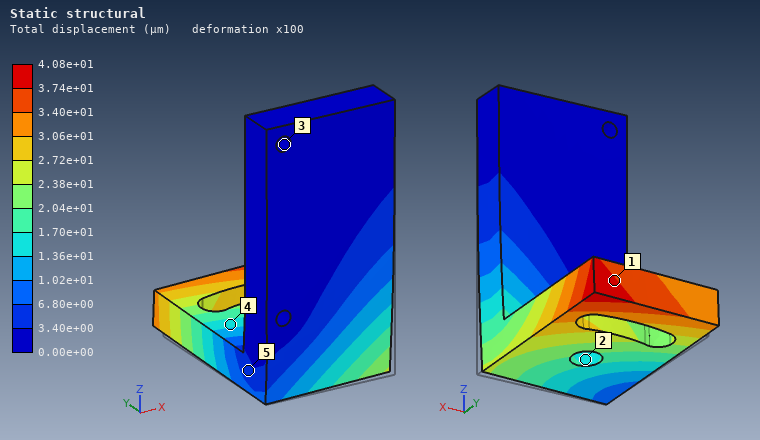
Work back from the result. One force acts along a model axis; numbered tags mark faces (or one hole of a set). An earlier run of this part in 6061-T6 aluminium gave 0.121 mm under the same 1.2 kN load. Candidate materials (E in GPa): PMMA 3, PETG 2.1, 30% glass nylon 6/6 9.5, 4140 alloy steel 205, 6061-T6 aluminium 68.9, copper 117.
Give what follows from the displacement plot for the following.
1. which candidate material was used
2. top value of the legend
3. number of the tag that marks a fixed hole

4140 alloy steel
4.08e+01 µm
3
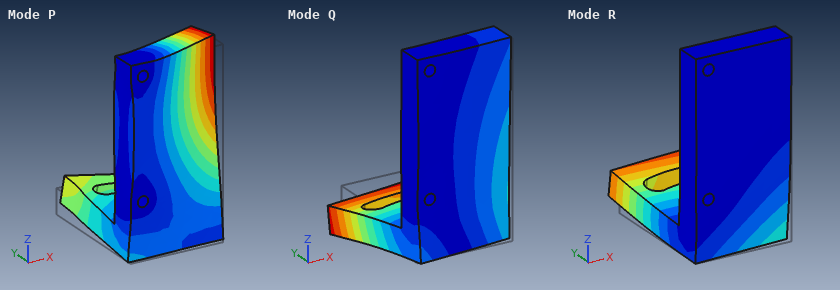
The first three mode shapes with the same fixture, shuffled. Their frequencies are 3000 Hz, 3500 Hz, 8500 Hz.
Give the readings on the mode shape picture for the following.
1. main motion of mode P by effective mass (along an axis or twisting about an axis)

along Y
